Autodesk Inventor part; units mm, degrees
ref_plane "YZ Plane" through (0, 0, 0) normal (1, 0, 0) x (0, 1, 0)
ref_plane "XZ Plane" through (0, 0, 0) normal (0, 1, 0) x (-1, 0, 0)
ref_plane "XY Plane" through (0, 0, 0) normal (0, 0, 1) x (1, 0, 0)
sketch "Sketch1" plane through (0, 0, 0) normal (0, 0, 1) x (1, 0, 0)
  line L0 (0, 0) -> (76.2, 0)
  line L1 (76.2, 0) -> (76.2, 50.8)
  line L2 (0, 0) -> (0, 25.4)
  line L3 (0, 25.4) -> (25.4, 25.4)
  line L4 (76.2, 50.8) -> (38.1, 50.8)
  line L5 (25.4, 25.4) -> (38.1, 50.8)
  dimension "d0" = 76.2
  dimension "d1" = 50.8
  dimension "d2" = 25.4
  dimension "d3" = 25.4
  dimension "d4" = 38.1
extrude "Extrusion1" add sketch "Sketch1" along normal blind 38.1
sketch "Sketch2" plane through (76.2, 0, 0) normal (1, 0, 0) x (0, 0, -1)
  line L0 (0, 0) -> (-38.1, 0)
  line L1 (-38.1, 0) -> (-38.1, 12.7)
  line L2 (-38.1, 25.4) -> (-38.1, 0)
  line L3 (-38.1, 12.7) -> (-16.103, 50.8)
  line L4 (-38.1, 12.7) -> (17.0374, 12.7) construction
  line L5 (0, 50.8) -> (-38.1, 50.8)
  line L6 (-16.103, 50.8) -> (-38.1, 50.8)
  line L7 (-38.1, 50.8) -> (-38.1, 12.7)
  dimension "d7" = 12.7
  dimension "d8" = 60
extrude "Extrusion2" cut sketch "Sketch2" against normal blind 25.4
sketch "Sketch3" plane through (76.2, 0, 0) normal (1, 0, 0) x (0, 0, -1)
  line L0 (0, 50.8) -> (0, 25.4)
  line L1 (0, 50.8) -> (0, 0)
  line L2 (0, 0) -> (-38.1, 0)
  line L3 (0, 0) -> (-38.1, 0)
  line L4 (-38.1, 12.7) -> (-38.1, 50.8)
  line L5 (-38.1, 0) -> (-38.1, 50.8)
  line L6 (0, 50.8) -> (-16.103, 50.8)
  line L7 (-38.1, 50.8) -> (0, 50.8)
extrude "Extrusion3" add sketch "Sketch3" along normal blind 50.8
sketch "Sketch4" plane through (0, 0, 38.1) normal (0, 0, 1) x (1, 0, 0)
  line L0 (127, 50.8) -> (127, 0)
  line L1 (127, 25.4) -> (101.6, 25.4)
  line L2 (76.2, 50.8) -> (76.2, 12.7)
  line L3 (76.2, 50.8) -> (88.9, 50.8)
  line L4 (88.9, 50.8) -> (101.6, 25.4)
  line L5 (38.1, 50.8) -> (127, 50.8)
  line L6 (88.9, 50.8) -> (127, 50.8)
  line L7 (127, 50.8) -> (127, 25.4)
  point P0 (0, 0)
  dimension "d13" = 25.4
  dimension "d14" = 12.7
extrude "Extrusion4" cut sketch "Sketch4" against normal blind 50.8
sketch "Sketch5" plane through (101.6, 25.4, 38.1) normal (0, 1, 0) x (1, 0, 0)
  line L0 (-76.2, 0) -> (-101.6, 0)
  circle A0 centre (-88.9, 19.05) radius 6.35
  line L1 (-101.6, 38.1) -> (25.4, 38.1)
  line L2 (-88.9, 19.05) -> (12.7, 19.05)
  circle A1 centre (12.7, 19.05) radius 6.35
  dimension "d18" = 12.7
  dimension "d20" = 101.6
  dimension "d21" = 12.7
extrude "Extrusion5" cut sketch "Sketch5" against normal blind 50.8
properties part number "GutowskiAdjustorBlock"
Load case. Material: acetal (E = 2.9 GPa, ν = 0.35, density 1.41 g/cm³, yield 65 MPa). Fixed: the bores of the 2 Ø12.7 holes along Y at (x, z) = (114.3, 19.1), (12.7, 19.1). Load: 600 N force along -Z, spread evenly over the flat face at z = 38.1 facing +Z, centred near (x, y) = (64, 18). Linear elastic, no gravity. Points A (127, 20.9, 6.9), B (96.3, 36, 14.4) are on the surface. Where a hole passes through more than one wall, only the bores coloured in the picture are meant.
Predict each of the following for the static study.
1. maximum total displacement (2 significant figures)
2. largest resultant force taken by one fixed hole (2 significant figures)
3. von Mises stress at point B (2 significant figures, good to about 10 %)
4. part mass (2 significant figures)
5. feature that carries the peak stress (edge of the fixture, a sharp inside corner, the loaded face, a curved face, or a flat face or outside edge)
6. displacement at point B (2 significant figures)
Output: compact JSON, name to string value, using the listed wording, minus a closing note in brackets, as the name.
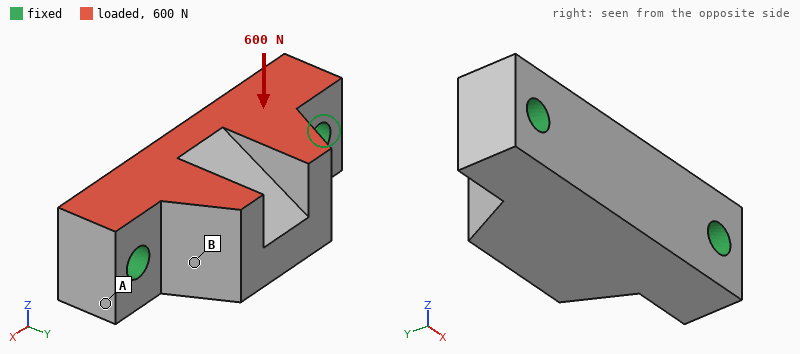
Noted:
{"maximum total displacement": "23 µm", "largest resultant force taken by one fixed hole": "300 N", "von Mises stress at point B": "0.33 MPa", "part mass": "240 g", "feature that carries the peak stress": "edge of the fixture", "displacement at point B": "13 µm"}
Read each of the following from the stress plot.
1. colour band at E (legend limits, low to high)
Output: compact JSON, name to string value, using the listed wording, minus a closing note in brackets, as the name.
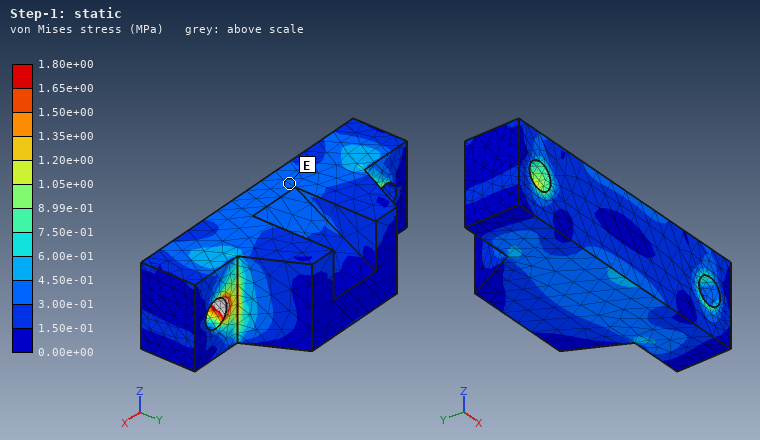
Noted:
{"colour band at E": "3.00e-01 to 4.50e-01 MPa"}
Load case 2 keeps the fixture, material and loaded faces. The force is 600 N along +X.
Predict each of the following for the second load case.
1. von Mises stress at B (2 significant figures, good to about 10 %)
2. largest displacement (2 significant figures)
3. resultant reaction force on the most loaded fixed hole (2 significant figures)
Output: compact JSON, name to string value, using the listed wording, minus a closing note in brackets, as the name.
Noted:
{"von Mises stress at B": "0.16 MPa", "largest displacement": "11 µm", "resultant reaction force on the most loaded fixed hole": "320 N"}
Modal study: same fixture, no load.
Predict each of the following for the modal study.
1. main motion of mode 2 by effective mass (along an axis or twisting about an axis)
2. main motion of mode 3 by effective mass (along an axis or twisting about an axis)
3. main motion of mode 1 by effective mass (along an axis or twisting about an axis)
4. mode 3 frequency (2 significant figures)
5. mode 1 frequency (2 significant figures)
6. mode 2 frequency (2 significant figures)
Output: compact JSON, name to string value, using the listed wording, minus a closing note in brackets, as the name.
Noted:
{"main motion of mode 2 by effective mass": "along Y", "main motion of mode 3 by effective mass": "along Z", "main motion of mode 1 by effective mass": "along Z", "mode 3 frequency": "3000 Hz", "mode 1 frequency": "1800 Hz", "mode 2 frequency": "2700 Hz"}
